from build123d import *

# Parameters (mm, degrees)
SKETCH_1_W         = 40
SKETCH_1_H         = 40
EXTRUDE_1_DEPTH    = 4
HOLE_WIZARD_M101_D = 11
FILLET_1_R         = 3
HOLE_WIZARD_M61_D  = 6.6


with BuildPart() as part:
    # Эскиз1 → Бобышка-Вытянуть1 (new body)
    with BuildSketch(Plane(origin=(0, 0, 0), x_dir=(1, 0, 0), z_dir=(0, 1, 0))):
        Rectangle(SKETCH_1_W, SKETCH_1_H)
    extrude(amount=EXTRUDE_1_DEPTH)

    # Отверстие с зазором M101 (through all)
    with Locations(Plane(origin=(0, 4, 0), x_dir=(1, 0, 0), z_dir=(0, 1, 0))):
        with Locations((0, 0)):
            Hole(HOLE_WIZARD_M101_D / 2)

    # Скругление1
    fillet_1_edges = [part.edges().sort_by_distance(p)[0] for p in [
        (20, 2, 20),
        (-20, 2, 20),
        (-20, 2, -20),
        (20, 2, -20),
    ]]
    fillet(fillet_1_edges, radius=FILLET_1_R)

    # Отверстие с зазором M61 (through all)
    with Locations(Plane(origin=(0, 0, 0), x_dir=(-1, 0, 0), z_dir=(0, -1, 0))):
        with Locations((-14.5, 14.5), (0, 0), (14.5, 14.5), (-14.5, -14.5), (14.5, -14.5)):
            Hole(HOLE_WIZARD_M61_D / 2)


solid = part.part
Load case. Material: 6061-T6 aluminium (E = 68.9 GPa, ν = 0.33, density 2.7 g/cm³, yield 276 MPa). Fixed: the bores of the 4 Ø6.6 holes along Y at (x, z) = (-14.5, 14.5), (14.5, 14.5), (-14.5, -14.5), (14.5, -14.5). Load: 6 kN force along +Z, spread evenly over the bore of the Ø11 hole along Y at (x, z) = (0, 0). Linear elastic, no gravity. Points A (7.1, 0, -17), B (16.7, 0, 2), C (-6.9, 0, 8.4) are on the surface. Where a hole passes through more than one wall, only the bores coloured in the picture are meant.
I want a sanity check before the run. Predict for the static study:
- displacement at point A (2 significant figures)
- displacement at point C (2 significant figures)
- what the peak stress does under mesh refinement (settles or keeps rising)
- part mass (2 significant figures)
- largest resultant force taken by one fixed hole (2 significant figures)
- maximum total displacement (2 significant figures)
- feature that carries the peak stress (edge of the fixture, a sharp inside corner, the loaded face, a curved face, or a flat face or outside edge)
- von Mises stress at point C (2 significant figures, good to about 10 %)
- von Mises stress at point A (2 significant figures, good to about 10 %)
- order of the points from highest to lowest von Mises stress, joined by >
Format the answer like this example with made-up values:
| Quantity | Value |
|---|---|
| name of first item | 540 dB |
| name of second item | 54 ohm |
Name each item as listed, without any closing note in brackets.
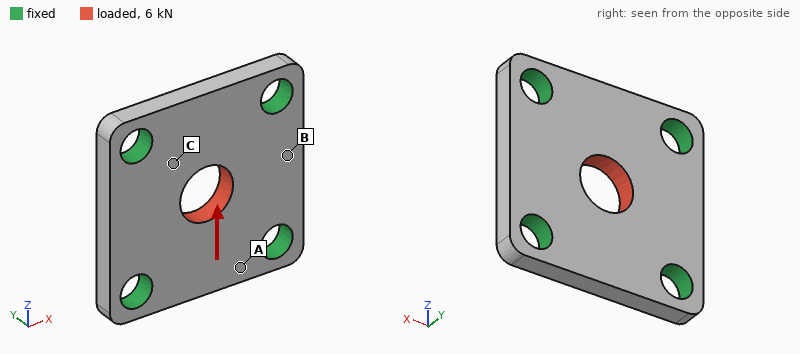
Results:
| Quantity | Value |
|---|---|
| displacement at point A | 4.3 µm |
| displacement at point C | 5.4 µm |
| what the peak stress does under mesh refinement | keeps rising |
| part mass | 15 g |
| largest resultant force taken by one fixed hole | 1.7 kN |
| maximum total displacement | 11 µm |
| feature that carries the peak stress | edge of the fixture |
| von Mises stress at point C | 39 MPa |
| von Mises stress at point A | 21 MPa |
| order of the points from highest to lowest von Mises stress, joined by > | C > A > B |
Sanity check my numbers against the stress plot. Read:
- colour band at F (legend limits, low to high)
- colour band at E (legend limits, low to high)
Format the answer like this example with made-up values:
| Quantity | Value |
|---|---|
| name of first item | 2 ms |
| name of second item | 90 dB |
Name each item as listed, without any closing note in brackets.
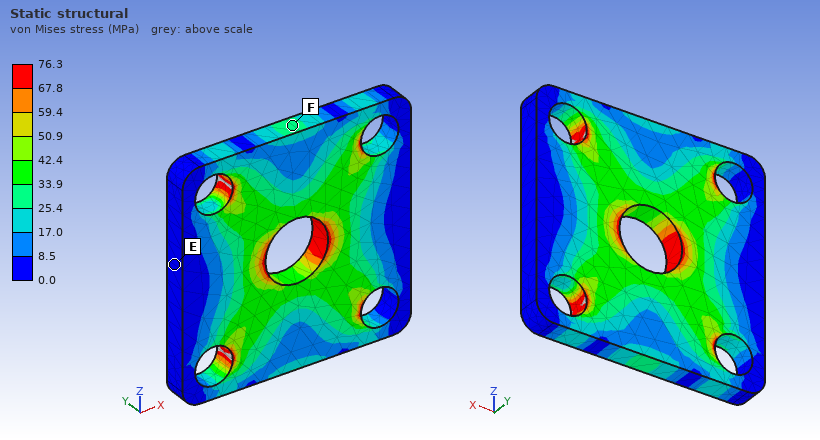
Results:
| Quantity | Value |
|---|---|
| colour band at F | 25.4 to 33.9 MPa |
| colour band at E | 0.0 to 8.5 MPa |
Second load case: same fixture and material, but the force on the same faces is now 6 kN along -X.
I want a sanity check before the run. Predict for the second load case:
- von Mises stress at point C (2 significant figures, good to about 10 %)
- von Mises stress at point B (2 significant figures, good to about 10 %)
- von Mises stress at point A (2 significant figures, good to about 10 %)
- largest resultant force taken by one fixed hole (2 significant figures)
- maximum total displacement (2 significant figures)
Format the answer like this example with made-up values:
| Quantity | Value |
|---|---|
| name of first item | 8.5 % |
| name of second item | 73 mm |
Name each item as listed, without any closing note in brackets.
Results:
| Quantity | Value |
|---|---|
| von Mises stress at point C | 38 MPa |
| von Mises stress at point B | 12 MPa |
| von Mises stress at point A | 8.7 MPa |
| largest resultant force taken by one fixed hole | 1.7 kN |
| maximum total displacement | 11 µm |
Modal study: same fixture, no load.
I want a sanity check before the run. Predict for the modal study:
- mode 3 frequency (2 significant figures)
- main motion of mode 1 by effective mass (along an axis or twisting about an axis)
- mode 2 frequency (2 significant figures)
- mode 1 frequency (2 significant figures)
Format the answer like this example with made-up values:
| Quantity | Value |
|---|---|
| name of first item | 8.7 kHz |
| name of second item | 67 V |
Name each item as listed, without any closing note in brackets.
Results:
| Quantity | Value |
|---|---|
| mode 3 frequency | 31 kHz |
| main motion of mode 1 by effective mass | along Y |
| mode 2 frequency | 31 kHz |
| mode 1 frequency | 23 kHz |
